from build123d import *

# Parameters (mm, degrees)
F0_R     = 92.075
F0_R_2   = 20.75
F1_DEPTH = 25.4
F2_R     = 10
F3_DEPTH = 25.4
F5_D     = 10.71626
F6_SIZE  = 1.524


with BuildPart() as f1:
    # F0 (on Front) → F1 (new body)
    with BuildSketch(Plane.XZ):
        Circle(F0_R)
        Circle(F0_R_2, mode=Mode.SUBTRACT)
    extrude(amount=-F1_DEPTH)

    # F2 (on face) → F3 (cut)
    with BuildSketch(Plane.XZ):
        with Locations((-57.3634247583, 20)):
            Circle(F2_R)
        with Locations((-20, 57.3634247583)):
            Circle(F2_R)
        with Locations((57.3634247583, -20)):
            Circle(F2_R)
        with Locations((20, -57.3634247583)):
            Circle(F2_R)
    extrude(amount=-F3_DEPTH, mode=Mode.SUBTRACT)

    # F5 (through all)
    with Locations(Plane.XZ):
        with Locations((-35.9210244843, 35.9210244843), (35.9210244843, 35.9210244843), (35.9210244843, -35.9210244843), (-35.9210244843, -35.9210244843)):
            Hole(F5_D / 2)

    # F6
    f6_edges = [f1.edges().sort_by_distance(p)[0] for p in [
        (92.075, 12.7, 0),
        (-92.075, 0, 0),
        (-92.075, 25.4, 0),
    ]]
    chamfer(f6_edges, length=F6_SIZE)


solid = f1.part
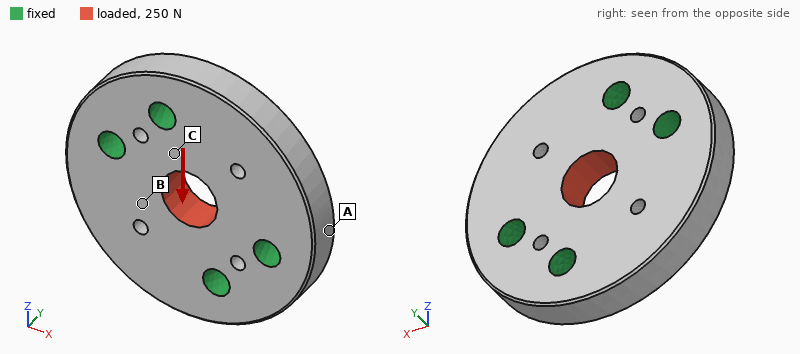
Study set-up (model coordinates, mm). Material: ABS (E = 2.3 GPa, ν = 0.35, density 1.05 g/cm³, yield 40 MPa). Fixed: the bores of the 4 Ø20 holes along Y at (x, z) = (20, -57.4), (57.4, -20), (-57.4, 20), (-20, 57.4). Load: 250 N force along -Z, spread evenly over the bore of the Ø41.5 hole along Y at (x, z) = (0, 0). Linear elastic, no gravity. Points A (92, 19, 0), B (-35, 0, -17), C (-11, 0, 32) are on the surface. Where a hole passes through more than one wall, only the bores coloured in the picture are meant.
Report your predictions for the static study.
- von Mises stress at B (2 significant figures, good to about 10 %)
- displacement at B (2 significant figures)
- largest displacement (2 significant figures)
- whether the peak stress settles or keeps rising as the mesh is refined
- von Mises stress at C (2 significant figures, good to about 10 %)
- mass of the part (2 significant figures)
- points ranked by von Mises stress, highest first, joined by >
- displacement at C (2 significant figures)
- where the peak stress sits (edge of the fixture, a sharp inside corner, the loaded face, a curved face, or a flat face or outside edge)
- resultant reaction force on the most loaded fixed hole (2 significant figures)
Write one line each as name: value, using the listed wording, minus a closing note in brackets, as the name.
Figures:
von Mises stress at B: 0.041 MPa
displacement at B: 1.0 µm
largest displacement: 1.8 µm
whether the peak stress settles or keeps rising as the mesh is refined: keeps rising
von Mises stress at C: 0.090 MPa
mass of the part: 630 g
points ranked by von Mises stress, highest first, joined by >: C > B > A
displacement at C: 0.87 µm
where the peak stress sits: edge of the fixture
resultant reaction force on the most loaded fixed hole: 80 N
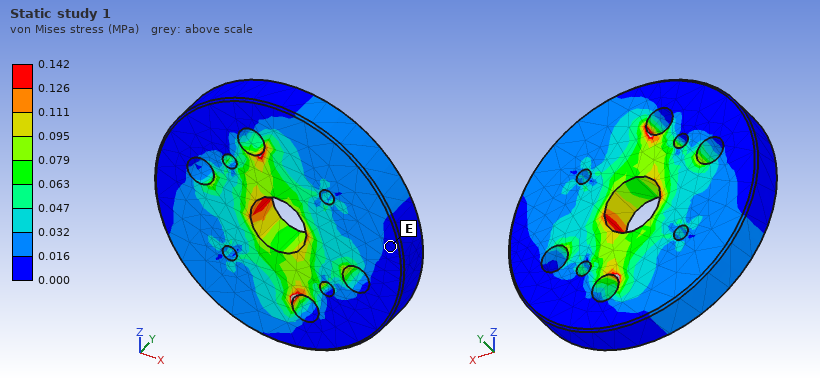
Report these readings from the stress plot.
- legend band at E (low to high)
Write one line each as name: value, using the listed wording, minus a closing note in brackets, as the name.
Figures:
legend band at E: 0.000 to 0.016 MPa
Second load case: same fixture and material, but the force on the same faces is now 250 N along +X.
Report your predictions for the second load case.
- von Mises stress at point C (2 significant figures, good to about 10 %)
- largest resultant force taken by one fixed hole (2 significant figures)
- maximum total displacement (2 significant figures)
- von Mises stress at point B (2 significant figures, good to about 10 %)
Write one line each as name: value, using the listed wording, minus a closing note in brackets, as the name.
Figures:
von Mises stress at point C: 0.052 MPa
largest resultant force taken by one fixed hole: 80 N
maximum total displacement: 1.8 µm
von Mises stress at point B: 0.052 MPa
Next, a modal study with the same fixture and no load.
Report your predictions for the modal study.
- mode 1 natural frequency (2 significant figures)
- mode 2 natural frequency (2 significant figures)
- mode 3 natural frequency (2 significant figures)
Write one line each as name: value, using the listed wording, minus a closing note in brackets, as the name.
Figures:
mode 1 natural frequency: 1400 Hz
mode 2 natural frequency: 1400 Hz
mode 3 natural frequency: 2900 Hz
